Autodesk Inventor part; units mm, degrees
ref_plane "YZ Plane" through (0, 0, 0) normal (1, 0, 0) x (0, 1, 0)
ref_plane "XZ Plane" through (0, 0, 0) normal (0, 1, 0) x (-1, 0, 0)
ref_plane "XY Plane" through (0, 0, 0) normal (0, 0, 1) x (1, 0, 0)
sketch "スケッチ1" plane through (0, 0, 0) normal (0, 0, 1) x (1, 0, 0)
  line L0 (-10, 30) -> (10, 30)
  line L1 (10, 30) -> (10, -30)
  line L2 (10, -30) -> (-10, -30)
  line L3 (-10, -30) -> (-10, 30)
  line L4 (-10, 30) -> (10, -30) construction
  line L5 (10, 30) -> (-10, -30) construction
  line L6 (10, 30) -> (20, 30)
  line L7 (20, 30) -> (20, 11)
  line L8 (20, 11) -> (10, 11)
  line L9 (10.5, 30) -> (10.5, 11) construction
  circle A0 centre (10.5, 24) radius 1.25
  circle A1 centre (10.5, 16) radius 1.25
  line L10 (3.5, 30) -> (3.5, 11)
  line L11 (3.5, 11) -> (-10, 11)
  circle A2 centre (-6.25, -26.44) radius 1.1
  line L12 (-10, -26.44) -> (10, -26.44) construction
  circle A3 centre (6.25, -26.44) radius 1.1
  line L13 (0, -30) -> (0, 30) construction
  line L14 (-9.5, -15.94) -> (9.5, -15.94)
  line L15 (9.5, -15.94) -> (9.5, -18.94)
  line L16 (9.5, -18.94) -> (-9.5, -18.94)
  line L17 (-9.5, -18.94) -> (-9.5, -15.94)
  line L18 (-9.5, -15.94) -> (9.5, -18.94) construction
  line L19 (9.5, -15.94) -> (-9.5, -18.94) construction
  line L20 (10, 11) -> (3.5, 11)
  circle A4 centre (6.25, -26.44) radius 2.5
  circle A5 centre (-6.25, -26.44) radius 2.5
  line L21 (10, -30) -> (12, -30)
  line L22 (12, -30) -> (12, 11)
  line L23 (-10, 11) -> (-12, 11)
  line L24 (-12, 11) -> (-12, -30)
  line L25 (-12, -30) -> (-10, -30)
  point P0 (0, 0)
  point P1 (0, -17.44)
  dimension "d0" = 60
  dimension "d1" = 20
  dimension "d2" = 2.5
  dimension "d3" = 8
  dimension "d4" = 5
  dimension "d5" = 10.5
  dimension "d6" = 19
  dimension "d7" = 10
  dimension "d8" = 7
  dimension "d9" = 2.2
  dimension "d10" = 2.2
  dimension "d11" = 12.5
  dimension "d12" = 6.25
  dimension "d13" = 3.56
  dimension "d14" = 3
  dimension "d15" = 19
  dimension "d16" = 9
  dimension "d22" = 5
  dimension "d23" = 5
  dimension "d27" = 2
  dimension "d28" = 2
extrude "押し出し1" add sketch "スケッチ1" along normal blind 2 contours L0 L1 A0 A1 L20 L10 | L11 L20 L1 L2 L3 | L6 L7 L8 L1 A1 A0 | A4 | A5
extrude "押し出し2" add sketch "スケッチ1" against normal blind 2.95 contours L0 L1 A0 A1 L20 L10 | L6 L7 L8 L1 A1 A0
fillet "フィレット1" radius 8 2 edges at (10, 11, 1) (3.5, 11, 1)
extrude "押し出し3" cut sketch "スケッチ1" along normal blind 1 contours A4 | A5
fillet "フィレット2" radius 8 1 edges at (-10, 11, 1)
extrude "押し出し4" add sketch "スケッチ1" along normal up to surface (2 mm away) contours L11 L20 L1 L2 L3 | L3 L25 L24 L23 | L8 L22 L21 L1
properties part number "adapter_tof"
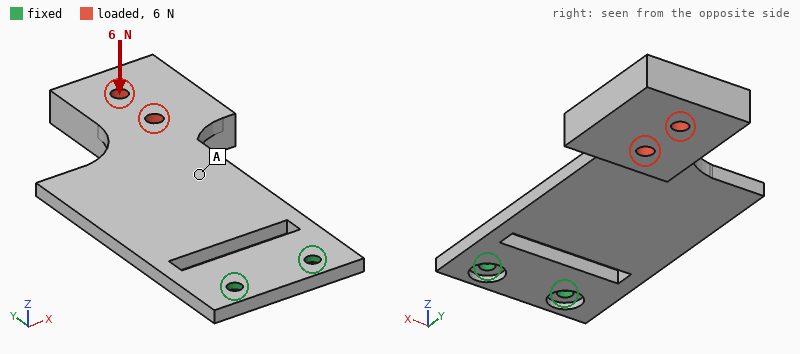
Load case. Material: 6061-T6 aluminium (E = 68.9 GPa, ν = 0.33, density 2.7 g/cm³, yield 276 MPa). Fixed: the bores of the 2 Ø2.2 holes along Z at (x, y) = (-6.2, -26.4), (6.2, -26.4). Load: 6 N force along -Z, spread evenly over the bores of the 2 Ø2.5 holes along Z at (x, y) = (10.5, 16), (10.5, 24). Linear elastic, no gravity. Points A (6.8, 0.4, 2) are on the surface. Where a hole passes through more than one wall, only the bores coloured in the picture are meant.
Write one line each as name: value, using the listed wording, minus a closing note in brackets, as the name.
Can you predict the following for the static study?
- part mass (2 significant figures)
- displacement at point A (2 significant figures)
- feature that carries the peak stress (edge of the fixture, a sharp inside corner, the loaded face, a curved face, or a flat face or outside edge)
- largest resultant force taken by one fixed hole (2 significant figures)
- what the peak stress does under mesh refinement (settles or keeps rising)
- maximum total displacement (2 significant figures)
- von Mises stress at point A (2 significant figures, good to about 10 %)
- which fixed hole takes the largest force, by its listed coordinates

part mass: 9.0 g
displacement at point A: 0.22 mm
feature that carries the peak stress: edge of the fixture
largest resultant force taken by one fixed hole: 7.9 N
what the peak stress does under mesh refinement: keeps rising
maximum total displacement: 0.63 mm
von Mises stress at point A: 9.4 MPa
which fixed hole takes the largest force, by its listed coordinates: (6.2, -26.4)
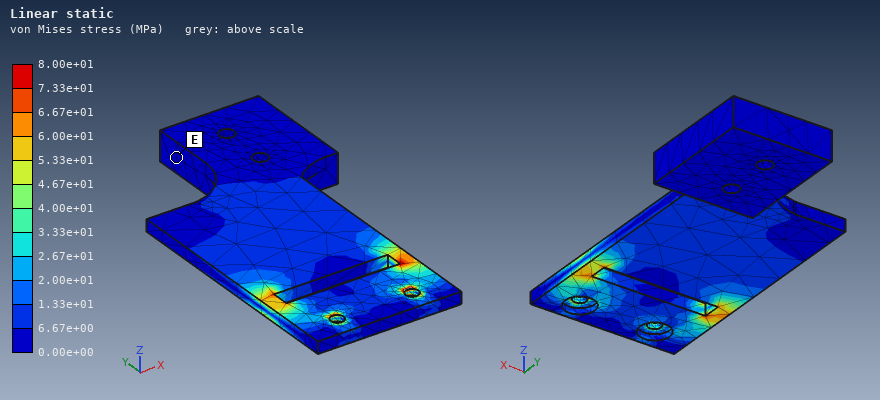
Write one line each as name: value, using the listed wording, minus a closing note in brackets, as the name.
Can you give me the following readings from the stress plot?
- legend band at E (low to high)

legend band at E: 0.00e+00 to 6.67e+00 MPa
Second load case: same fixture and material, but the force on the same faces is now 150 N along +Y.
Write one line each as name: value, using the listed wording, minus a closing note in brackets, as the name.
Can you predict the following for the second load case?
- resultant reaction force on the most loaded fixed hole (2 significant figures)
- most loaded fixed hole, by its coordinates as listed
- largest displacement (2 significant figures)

resultant reaction force on the most loaded fixed hole: 190 N
most loaded fixed hole, by its coordinates as listed: (6.2, -26.4)
largest displacement: 0.68 mm
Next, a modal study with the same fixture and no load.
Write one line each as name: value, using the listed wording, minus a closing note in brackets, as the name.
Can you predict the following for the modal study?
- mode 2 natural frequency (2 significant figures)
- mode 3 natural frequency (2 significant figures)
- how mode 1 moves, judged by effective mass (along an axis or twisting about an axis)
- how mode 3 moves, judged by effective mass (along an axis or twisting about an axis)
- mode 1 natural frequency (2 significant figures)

mode 2 natural frequency: 1800 Hz
mode 3 natural frequency: 2500 Hz
how mode 1 moves, judged by effective mass: along Z
how mode 3 moves, judged by effective mass: along X
mode 1 natural frequency: 250 Hz
